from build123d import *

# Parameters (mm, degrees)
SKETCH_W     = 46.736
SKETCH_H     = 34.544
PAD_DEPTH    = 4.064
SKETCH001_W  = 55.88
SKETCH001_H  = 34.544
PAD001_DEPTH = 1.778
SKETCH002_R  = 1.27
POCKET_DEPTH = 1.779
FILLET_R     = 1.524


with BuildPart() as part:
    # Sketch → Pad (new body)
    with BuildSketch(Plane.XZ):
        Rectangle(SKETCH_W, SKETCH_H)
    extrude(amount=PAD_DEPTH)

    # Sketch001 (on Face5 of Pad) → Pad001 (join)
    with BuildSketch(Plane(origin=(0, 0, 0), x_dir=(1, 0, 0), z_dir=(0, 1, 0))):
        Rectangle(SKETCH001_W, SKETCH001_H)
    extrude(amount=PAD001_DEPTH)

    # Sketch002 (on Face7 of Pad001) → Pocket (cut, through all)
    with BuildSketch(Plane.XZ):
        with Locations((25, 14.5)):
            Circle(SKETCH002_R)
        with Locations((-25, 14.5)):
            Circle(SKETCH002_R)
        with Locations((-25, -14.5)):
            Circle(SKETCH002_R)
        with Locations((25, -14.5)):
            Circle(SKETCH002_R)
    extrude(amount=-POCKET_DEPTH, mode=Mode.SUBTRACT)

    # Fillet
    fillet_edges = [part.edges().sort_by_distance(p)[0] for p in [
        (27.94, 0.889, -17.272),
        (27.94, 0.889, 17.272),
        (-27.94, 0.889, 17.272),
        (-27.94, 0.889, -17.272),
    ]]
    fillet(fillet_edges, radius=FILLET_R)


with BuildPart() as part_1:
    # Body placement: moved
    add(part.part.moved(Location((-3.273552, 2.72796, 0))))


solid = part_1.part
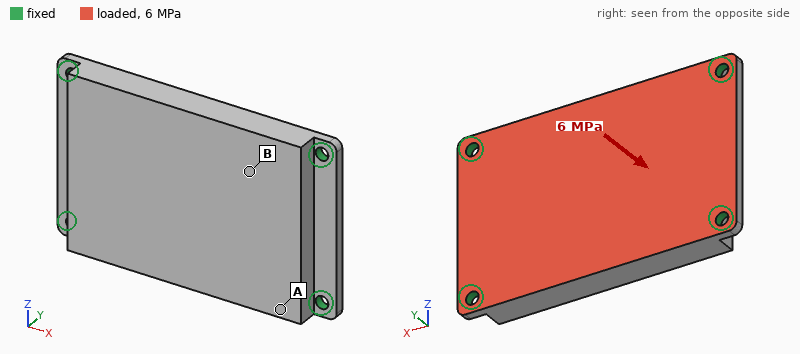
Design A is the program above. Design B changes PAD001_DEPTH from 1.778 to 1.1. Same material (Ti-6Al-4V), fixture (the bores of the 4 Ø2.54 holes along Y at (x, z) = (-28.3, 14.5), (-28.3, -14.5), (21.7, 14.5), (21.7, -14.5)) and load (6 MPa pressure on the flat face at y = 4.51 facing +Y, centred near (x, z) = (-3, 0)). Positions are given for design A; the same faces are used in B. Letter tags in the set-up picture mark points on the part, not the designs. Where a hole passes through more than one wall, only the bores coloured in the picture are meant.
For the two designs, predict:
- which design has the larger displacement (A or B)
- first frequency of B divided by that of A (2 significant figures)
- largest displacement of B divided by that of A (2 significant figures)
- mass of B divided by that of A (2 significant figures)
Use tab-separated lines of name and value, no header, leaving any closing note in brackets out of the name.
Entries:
which design has the larger displacement	B
first frequency of B divided by that of A	0.89
largest displacement of B divided by that of A	1.4
mass of B divided by that of A	0.87
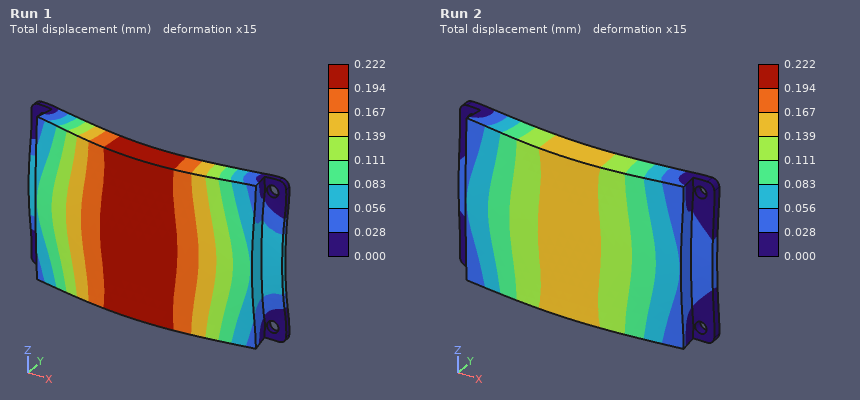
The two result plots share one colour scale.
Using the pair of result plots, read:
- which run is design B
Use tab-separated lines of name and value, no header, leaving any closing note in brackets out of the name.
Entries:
which run is design B	Run 1
